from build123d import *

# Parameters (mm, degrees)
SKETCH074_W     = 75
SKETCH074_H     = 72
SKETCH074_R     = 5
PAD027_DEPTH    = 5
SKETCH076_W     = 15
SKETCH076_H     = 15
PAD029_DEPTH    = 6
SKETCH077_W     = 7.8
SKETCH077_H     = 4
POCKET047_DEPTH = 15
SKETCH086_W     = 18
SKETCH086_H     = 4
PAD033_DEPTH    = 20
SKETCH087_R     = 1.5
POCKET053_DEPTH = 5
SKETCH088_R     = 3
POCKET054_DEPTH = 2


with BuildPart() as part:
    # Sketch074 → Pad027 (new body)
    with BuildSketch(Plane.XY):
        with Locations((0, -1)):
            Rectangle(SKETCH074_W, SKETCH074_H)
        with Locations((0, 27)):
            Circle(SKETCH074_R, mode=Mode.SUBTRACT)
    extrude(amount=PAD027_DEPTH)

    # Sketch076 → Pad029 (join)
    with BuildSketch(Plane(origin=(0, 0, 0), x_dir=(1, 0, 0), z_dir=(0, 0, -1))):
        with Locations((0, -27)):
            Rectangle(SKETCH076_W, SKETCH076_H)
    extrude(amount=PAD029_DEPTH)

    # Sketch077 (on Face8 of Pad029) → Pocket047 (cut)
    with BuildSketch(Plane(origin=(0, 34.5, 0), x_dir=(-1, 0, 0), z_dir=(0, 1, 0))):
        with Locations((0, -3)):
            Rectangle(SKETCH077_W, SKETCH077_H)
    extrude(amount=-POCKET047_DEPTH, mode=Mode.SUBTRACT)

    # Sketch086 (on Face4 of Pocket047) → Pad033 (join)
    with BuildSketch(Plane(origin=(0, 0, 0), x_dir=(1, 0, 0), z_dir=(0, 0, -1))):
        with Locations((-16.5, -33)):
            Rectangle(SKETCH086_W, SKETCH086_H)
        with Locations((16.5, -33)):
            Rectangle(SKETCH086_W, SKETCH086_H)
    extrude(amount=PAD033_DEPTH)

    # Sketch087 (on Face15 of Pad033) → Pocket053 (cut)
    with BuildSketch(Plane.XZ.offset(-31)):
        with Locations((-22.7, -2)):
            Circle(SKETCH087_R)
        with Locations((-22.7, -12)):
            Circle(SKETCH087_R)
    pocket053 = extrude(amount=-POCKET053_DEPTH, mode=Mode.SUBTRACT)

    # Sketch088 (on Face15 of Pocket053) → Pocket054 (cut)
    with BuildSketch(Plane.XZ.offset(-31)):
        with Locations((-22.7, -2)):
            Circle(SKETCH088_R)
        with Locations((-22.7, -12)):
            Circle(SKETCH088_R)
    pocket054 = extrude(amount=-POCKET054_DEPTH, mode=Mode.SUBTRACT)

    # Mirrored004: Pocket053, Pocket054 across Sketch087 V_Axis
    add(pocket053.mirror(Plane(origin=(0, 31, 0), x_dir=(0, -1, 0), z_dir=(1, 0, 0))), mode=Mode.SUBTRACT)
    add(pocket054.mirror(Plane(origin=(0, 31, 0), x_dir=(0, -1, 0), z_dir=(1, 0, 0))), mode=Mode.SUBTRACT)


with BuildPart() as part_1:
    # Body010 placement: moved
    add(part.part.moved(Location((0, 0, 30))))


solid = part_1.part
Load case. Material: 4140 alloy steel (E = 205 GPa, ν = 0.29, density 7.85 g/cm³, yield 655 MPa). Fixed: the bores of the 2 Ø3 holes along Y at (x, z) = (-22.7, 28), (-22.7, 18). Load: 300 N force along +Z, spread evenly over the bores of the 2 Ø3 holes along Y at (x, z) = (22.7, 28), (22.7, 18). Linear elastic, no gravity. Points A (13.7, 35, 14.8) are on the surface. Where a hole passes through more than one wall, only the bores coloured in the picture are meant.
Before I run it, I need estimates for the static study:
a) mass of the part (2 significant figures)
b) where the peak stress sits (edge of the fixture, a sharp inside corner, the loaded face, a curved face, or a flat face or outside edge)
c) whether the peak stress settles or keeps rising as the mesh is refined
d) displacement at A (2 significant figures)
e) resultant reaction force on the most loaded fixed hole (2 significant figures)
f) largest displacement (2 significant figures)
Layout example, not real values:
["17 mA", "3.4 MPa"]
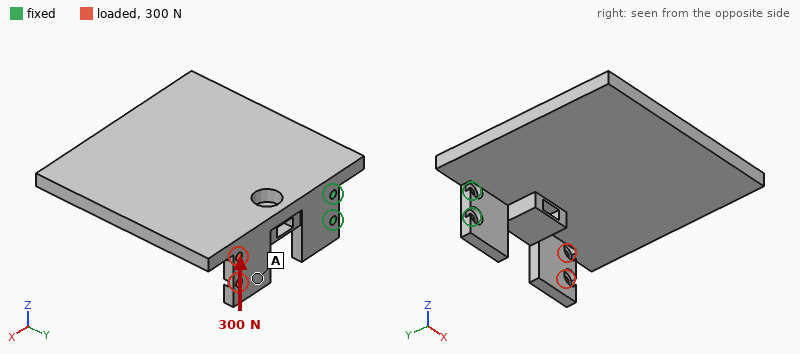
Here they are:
["240 g", "edge of the fixture", "keeps rising", "50 µm", "1.1 kN", "83 µm"]
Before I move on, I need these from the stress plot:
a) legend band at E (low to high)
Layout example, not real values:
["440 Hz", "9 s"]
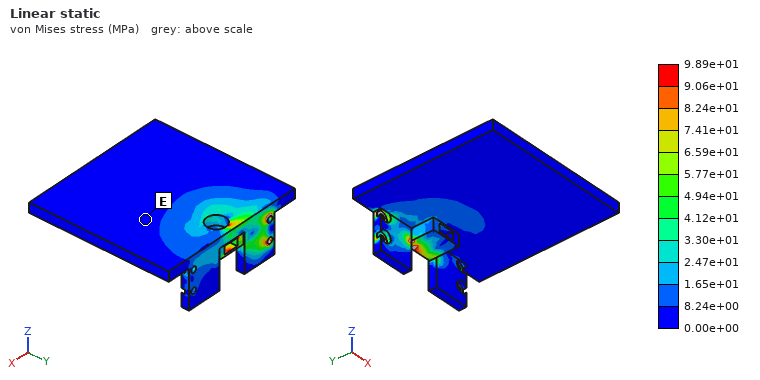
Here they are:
["0.00e+00 to 8.24e+00 MPa"]
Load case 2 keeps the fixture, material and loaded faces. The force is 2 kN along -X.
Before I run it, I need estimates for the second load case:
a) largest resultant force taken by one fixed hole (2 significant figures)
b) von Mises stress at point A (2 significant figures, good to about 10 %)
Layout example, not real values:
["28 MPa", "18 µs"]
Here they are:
["1.1 kN", "22 MPa"]
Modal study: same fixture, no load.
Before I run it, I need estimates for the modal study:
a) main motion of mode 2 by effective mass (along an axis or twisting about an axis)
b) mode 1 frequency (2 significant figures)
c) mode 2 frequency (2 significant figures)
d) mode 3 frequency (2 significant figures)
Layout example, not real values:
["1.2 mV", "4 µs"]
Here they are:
["along Z", "290 Hz", "410 Hz", "1100 Hz"]
